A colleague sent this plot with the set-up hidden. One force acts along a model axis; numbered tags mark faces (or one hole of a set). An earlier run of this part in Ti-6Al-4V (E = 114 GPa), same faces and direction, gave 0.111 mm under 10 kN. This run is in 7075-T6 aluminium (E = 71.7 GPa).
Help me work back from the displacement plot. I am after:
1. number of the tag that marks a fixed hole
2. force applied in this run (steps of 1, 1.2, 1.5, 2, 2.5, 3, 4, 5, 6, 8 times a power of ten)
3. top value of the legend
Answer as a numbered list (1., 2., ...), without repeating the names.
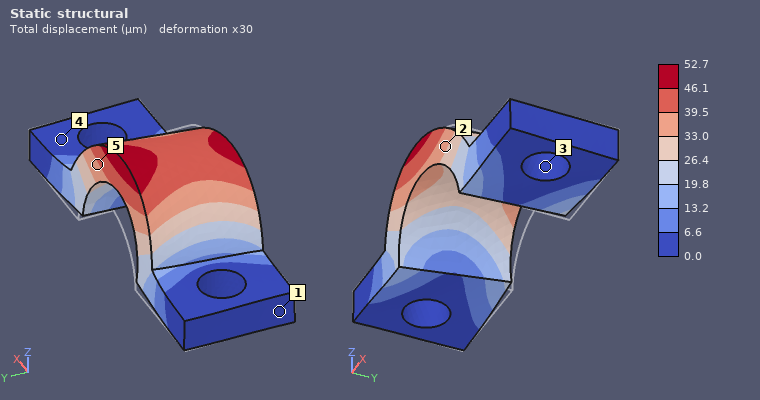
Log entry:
1. 3
2. 3 kN
3. 52.7 µm
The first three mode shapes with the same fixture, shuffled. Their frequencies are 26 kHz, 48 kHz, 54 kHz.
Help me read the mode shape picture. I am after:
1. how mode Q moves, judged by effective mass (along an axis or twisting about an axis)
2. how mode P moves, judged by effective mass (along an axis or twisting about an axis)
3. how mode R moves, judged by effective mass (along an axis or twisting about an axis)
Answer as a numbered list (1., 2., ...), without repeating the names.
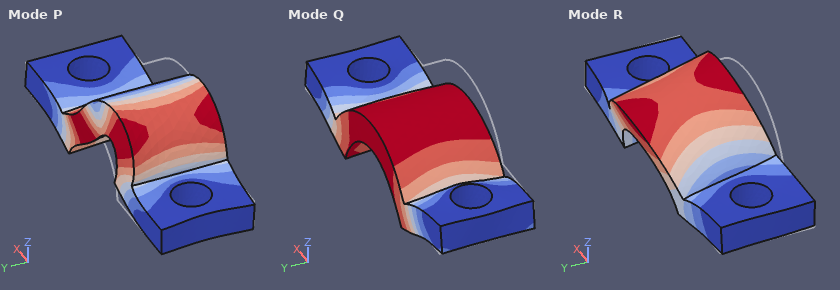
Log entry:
1. along Z
2. along X
3. along Y
